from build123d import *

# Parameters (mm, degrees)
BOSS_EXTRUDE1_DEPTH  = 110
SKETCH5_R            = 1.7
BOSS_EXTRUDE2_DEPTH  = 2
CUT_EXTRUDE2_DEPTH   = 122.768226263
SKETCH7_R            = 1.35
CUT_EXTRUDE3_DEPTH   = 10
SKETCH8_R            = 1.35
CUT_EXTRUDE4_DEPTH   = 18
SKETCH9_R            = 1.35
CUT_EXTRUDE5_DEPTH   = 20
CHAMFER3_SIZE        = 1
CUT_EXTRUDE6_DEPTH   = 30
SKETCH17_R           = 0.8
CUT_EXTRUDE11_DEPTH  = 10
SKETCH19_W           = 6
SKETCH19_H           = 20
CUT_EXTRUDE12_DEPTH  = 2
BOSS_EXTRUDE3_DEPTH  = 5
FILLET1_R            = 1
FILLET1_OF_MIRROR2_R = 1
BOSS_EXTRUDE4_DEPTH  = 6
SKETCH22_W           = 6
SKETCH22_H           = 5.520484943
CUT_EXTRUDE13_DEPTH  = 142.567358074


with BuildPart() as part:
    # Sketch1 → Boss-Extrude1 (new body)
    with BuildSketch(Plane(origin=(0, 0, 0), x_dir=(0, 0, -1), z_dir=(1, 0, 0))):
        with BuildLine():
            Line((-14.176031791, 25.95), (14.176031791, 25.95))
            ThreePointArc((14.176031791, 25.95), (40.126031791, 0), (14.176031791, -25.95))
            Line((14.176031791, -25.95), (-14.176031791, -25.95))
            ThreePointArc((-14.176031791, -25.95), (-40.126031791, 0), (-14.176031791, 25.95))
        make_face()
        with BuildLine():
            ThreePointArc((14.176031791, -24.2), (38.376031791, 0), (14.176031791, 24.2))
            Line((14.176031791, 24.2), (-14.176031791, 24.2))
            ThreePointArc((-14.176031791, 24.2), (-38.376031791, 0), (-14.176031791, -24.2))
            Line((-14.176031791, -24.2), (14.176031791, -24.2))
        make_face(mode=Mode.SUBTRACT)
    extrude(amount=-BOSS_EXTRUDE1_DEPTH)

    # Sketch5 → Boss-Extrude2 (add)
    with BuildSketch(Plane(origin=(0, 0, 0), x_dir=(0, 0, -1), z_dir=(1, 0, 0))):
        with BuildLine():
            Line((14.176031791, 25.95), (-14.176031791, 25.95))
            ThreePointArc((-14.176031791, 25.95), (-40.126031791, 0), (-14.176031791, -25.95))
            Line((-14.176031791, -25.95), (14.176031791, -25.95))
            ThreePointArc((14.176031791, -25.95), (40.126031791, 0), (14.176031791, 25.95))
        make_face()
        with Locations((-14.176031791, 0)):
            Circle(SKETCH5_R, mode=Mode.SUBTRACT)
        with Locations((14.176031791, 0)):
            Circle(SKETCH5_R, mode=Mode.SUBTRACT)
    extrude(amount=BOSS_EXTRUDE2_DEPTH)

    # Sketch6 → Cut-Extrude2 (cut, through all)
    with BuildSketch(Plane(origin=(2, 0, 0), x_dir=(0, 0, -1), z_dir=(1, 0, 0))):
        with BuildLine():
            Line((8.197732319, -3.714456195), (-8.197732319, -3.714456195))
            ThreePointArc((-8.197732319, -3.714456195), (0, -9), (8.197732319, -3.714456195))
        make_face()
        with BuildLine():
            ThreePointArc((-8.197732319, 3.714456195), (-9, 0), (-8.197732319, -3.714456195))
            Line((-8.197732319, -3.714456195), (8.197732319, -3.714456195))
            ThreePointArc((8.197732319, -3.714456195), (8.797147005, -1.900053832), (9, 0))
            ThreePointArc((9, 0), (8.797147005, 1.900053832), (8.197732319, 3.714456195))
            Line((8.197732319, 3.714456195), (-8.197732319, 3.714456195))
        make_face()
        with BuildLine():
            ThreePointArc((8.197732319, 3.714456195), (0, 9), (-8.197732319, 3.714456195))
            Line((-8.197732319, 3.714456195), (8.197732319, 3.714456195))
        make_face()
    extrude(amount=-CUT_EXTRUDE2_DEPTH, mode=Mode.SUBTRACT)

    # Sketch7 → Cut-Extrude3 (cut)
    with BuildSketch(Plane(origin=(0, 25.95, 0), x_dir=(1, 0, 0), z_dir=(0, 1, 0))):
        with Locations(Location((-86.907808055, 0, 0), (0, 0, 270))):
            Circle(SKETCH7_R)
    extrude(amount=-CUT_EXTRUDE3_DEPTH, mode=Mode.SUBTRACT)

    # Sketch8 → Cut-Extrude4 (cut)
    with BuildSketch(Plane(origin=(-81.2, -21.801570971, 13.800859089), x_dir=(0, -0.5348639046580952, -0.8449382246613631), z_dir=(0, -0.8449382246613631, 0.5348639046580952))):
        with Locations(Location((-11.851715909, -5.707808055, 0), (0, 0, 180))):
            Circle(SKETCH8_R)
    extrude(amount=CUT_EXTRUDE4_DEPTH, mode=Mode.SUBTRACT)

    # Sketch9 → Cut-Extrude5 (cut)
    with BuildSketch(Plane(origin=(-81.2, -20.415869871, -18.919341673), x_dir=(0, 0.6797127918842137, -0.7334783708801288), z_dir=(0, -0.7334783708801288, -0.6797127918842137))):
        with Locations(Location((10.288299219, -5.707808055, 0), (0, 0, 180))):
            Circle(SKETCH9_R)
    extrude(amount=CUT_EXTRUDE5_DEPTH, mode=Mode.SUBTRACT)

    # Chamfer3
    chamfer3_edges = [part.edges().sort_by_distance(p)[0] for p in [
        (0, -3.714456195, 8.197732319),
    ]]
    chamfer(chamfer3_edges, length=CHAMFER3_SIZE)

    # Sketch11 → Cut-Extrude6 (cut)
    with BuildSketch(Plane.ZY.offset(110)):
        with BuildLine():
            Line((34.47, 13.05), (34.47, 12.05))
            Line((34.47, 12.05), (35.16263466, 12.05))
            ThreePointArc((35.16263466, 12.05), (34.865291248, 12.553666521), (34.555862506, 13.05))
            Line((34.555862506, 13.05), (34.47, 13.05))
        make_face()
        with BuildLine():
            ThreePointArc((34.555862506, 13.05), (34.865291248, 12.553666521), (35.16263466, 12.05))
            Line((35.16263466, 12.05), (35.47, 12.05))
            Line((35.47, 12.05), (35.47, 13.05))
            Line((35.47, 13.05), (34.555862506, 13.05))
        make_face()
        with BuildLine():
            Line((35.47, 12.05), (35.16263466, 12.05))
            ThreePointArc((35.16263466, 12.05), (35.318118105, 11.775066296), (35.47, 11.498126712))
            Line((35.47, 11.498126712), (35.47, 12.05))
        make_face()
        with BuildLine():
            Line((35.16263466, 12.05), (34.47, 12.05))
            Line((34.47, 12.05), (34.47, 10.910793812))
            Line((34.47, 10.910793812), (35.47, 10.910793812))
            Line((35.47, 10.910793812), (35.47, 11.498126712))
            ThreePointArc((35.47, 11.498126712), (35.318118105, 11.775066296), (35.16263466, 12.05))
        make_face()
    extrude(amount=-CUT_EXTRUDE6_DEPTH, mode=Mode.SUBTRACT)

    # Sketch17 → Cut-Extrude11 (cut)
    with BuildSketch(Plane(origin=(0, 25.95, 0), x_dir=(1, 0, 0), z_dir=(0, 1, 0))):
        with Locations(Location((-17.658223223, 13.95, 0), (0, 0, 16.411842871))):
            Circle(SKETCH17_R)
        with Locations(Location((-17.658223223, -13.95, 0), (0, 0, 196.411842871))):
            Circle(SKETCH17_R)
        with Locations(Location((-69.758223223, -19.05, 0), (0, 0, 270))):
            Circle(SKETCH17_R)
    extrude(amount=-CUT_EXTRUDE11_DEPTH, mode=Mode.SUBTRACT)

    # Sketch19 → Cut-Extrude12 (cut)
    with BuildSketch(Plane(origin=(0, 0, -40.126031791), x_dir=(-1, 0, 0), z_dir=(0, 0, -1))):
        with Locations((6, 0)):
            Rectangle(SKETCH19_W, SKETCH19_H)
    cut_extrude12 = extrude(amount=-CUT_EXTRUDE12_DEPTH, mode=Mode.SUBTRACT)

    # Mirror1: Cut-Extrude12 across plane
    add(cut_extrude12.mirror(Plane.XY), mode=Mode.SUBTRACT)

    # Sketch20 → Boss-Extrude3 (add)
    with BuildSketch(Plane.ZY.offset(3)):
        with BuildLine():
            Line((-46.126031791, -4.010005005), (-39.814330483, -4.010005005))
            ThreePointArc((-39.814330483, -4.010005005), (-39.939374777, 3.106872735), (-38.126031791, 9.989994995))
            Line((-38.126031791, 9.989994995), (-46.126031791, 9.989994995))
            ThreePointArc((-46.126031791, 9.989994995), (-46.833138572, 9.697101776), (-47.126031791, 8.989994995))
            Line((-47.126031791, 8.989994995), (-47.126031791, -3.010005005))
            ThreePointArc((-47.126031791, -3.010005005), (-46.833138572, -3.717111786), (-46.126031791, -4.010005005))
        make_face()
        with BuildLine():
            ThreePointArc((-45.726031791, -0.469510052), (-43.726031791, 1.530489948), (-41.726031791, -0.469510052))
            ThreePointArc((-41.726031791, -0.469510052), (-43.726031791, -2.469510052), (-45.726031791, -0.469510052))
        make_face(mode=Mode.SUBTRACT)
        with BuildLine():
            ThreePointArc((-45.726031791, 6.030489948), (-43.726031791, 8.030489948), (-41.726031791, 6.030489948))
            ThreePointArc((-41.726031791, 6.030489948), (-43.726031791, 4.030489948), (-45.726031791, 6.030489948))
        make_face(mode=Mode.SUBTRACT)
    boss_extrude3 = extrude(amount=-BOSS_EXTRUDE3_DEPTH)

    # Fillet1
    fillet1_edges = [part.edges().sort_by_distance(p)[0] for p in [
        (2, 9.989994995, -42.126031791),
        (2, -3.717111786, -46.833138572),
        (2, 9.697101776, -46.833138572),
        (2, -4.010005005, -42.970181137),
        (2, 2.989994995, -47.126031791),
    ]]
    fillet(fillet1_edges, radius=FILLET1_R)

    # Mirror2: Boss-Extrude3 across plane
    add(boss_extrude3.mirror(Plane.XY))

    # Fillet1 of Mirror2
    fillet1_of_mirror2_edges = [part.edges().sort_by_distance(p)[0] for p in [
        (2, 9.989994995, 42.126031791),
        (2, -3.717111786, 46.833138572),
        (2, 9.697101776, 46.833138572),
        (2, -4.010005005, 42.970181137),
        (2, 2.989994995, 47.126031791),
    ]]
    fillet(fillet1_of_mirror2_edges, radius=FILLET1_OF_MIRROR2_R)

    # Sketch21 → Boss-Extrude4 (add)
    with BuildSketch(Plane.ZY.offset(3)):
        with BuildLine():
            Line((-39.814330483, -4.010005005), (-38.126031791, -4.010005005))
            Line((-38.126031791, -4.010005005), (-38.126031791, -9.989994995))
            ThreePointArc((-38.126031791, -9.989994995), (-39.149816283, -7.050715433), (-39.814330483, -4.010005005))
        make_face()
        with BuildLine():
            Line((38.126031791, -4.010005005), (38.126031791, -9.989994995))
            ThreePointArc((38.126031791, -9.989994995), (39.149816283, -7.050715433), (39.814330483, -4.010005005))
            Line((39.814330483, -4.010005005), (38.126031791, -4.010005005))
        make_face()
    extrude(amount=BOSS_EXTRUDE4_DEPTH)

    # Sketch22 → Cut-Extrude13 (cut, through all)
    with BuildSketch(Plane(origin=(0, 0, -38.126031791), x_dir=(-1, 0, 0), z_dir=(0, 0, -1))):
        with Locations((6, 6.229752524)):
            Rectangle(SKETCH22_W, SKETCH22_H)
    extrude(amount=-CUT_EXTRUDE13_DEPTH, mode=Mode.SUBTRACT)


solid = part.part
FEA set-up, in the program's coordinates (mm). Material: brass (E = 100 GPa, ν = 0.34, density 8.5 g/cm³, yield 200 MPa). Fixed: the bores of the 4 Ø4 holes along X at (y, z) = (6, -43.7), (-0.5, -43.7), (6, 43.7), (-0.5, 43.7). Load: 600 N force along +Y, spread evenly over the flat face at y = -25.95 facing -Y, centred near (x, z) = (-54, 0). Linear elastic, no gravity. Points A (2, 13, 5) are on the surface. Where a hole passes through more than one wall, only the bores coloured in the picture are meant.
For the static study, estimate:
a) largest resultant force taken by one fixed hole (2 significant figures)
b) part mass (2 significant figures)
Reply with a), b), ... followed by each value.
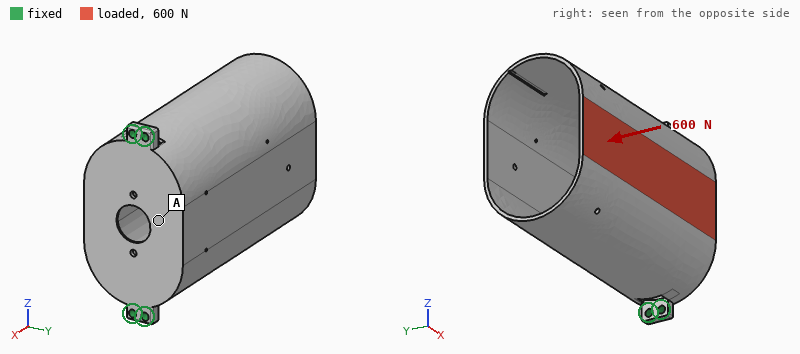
a) 1.3 kN
b) 410 g
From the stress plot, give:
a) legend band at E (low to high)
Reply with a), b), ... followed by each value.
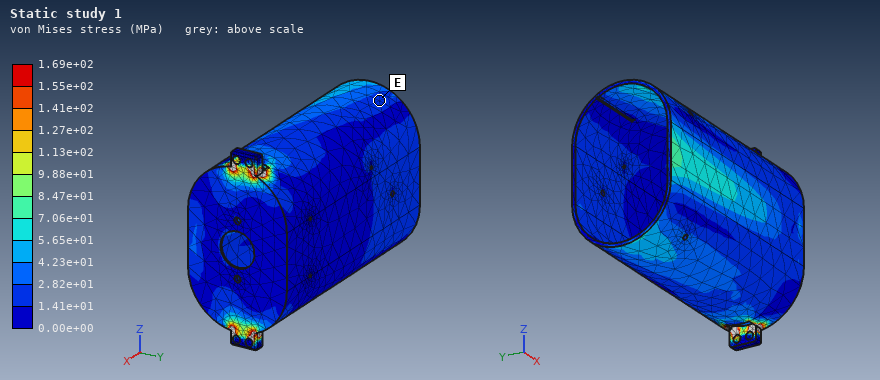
a) 1.41e+01 to 2.82e+01 MPa
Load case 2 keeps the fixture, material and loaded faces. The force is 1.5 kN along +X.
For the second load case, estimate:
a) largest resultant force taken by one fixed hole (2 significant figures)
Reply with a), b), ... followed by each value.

a) 2.1 kN
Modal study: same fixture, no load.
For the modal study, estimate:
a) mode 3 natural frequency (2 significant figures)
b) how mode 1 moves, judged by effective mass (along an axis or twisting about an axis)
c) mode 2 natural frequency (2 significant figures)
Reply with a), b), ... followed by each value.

a) 730 Hz
b) along Y
c) 690 Hz
